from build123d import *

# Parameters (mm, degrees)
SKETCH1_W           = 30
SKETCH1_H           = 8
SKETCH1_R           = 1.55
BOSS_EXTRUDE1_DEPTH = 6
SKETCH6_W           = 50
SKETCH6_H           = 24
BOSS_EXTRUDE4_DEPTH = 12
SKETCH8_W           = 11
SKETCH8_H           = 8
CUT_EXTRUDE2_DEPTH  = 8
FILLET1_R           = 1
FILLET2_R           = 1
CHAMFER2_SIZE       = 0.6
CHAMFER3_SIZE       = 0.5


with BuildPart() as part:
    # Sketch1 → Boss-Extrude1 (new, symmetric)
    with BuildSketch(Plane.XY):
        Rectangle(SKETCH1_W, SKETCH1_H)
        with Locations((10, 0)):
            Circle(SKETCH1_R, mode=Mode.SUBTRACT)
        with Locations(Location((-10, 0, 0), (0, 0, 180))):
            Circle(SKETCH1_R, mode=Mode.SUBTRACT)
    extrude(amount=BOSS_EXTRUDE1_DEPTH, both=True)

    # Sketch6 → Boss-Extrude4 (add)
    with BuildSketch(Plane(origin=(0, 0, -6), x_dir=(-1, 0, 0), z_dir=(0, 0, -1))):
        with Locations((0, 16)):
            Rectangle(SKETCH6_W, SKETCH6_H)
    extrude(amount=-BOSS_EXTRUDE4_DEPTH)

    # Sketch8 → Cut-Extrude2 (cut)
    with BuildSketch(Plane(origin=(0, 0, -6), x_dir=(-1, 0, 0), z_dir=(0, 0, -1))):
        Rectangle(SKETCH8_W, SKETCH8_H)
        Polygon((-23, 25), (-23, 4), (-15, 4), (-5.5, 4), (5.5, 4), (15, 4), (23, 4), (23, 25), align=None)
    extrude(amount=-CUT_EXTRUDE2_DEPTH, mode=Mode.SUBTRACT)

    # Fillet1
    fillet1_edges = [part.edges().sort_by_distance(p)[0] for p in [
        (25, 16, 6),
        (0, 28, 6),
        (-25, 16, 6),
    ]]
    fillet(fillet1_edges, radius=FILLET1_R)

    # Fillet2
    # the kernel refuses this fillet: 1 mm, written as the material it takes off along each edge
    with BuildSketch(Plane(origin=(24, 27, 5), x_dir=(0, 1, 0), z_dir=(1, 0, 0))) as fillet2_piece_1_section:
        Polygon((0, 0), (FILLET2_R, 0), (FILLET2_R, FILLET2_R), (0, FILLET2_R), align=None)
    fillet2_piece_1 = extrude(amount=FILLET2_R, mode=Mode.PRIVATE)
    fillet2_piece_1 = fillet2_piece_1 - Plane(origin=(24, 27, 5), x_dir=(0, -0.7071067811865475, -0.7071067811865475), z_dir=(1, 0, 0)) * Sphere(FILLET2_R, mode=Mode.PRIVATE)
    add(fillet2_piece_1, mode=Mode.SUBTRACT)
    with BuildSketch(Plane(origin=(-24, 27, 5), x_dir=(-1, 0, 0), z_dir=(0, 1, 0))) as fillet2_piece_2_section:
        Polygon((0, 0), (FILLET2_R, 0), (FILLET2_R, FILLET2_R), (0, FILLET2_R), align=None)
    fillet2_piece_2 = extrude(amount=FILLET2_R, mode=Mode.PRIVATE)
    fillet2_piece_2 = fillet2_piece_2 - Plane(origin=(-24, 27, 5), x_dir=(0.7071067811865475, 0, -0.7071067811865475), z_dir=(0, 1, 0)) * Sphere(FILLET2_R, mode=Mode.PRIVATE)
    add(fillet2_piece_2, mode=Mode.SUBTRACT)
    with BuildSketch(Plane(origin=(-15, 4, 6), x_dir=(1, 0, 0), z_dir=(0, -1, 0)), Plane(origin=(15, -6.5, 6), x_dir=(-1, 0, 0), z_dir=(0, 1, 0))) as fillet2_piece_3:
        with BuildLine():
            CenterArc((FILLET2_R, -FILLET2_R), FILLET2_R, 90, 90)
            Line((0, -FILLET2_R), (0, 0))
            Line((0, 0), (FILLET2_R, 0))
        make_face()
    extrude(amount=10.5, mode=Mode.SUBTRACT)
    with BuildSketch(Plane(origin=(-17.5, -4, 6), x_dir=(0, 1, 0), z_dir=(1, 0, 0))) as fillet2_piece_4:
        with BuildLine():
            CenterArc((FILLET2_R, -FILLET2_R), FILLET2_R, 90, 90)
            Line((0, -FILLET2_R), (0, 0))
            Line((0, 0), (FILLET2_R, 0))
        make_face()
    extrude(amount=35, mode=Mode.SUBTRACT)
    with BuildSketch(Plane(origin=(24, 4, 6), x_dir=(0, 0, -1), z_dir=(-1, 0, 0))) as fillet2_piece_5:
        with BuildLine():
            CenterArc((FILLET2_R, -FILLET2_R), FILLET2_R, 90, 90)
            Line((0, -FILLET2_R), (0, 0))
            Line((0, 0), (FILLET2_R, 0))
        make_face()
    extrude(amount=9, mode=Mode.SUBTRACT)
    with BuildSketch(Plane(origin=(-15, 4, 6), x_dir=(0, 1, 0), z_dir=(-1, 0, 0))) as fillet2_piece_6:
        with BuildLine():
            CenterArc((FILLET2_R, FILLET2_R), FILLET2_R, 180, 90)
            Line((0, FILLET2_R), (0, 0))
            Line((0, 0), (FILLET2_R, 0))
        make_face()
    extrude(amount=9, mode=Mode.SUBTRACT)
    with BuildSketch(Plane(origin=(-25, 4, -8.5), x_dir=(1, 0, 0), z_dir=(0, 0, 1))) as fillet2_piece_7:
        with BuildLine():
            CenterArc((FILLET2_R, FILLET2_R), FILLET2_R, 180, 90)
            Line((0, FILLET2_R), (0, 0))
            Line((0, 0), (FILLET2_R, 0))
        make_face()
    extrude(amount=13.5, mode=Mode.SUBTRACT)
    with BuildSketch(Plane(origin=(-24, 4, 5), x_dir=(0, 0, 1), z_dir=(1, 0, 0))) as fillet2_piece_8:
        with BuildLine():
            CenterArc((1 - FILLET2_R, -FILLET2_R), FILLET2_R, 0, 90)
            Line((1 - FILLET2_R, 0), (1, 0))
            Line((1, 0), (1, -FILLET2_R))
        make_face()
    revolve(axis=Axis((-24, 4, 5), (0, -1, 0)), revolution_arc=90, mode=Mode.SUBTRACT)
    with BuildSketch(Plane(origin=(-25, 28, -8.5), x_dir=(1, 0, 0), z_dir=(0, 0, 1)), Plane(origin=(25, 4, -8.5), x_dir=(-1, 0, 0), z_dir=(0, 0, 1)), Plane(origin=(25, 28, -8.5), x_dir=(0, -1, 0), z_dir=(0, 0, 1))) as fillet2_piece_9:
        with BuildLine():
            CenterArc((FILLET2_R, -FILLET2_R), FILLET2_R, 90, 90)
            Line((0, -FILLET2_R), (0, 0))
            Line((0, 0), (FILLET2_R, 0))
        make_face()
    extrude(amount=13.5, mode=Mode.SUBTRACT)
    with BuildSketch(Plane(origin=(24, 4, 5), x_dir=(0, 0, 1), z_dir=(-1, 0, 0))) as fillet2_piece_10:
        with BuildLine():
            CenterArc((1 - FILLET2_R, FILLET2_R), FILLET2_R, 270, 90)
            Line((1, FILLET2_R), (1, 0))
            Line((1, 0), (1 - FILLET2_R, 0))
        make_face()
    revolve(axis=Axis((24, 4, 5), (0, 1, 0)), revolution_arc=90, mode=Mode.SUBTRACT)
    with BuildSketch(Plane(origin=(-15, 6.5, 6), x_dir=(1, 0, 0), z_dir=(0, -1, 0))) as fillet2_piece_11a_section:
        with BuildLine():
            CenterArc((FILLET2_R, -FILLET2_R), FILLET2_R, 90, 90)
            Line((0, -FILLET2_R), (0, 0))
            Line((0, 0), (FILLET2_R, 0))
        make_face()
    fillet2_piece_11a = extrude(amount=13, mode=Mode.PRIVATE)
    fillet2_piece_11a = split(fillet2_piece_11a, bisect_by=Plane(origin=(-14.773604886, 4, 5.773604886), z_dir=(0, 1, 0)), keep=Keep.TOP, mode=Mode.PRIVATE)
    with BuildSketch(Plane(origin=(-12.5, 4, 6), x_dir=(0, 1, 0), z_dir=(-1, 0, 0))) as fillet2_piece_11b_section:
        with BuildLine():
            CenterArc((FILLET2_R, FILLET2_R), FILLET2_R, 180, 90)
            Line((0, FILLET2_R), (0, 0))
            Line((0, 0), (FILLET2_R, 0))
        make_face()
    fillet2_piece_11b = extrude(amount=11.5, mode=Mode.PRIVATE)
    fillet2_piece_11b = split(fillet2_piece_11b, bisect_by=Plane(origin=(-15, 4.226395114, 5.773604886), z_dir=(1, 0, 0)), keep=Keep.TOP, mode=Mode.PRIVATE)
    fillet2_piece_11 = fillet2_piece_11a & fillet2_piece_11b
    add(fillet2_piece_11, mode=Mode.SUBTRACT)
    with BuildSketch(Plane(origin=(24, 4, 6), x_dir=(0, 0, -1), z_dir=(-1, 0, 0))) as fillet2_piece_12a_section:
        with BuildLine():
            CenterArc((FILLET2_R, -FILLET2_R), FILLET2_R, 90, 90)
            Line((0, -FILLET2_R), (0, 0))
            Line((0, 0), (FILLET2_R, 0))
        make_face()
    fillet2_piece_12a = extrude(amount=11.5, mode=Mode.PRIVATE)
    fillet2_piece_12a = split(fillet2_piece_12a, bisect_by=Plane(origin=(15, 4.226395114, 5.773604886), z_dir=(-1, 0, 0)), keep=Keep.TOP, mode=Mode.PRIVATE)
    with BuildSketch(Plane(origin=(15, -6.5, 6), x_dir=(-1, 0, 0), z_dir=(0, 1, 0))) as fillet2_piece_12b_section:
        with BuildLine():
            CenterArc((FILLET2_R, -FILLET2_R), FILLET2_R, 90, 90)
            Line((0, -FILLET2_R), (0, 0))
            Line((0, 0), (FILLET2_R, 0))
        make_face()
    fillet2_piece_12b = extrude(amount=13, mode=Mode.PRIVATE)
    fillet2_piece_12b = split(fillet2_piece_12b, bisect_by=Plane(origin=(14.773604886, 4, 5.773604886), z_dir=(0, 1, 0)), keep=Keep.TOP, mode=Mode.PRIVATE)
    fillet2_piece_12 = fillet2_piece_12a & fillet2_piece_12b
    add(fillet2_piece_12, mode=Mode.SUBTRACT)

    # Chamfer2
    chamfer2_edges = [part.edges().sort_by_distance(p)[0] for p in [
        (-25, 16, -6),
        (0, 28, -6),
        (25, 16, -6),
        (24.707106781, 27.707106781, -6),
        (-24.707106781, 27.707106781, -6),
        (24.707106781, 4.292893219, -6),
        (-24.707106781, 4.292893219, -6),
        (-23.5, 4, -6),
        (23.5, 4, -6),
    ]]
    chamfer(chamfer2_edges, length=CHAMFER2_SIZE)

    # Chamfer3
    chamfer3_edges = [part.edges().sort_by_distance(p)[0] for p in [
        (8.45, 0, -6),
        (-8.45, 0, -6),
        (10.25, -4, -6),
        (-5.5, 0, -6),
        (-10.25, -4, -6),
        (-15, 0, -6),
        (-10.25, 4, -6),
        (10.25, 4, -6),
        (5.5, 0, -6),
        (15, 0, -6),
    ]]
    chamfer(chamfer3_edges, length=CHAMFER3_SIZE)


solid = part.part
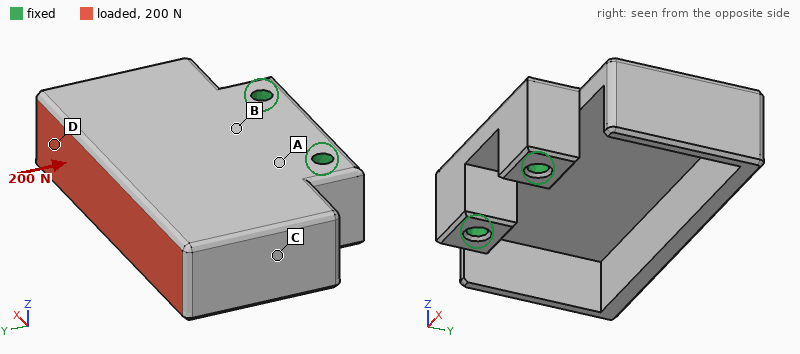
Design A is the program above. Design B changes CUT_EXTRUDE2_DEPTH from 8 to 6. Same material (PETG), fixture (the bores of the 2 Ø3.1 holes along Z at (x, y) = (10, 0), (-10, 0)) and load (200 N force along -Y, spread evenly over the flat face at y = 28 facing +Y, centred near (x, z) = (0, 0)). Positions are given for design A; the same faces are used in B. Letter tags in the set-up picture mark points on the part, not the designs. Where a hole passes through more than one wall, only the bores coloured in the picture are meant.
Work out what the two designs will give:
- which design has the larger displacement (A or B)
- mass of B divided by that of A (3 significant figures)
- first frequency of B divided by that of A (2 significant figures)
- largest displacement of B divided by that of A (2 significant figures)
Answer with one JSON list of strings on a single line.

["A", "1.25", "1.6", "0.27"]
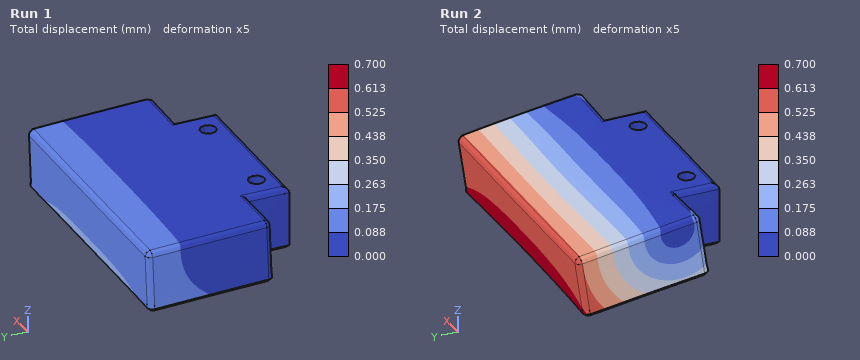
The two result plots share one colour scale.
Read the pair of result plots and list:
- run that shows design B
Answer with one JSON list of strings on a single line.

["Run 1"]
